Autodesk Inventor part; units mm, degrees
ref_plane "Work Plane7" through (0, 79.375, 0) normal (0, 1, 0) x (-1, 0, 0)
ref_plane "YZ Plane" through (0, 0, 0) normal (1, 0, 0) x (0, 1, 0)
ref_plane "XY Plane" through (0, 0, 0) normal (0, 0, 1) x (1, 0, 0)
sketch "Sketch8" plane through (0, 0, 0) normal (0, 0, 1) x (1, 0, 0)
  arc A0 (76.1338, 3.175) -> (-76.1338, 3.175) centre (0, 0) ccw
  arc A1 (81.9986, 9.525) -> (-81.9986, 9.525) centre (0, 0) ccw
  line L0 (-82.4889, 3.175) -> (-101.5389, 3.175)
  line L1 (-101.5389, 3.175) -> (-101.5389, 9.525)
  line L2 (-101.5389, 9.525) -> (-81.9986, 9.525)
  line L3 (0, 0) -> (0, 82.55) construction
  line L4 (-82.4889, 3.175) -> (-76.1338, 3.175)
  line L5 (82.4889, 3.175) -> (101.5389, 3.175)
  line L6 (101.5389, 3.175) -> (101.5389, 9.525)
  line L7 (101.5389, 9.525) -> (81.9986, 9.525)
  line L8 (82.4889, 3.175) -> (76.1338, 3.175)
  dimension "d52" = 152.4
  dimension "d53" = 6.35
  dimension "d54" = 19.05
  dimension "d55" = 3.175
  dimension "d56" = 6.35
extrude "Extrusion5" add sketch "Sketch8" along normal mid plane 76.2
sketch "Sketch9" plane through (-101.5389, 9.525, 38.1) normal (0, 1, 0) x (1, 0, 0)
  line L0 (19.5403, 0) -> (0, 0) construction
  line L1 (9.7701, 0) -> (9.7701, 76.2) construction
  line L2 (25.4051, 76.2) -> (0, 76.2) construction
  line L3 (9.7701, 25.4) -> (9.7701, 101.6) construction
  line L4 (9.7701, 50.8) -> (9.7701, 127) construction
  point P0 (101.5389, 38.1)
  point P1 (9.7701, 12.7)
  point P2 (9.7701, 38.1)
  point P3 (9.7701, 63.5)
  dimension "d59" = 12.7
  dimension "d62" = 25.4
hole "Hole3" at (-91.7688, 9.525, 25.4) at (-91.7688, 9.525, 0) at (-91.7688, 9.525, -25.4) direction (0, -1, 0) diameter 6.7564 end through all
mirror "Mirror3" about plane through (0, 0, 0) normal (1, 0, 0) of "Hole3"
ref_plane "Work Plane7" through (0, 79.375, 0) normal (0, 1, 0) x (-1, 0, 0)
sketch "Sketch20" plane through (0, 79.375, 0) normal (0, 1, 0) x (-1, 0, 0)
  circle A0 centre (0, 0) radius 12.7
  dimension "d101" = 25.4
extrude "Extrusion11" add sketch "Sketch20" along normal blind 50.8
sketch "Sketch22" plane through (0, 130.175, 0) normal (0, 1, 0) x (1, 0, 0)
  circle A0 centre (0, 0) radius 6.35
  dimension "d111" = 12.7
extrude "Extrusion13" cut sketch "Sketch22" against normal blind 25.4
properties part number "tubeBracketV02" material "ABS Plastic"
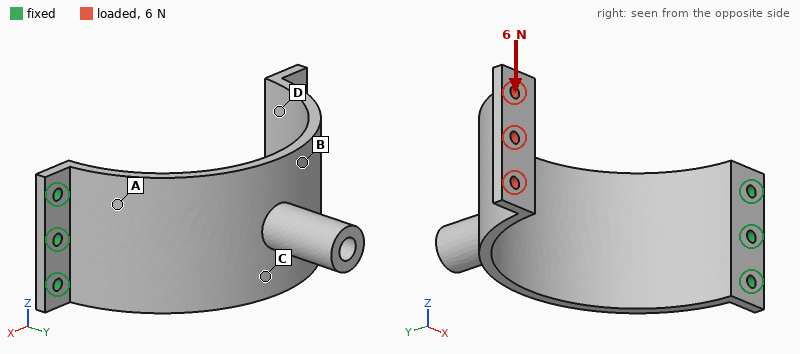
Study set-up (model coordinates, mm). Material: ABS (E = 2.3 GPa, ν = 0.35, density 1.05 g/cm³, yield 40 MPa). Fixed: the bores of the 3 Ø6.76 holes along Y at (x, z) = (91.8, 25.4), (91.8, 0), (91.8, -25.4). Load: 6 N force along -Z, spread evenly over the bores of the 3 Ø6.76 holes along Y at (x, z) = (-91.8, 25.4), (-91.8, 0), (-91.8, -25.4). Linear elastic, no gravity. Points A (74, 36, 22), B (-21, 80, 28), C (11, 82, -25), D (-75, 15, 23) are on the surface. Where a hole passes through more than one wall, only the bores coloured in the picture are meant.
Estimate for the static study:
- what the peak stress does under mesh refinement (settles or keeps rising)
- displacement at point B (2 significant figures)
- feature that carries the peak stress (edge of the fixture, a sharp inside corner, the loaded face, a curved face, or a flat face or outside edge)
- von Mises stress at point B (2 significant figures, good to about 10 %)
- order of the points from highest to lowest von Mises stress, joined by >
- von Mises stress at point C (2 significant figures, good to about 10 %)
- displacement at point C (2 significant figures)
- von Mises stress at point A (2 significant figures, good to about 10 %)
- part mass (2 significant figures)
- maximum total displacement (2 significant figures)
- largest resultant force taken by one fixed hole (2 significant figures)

keeps rising
0.70 mm
edge of the fixture
0.39 MPa
A > C > B > D
0.77 MPa
0.42 mm
1.3 MPa
160 g
2.3 mm
20 N
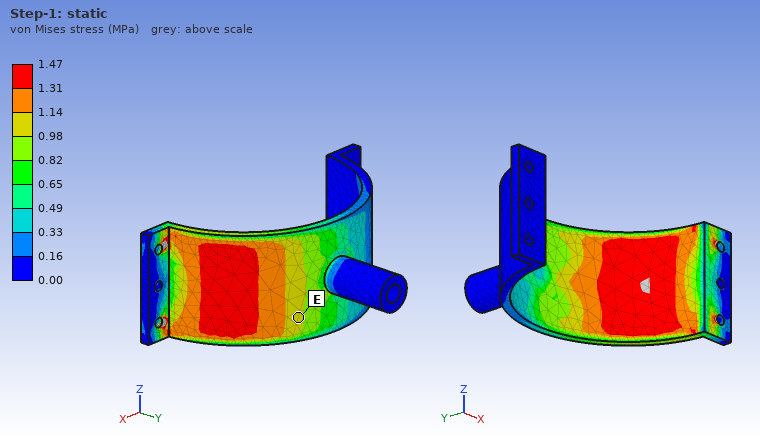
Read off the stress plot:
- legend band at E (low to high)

0.98 to 1.14 MPa
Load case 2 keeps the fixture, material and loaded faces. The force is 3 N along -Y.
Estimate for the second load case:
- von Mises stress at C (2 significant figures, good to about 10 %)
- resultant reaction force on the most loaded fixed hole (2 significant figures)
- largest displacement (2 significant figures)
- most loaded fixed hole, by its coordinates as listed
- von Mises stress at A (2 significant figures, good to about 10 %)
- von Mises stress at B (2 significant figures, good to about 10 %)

0.44 MPa
4.8 N
2.5 mm
(91.8, 0)
0.84 MPa
0.36 MPa
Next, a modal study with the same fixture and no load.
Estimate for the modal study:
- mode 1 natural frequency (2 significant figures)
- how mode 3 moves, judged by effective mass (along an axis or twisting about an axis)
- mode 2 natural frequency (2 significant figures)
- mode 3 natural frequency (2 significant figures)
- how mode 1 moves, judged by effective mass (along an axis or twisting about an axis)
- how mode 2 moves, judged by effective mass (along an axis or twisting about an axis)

26 Hz
along X
46 Hz
83 Hz
along Y
along Z
